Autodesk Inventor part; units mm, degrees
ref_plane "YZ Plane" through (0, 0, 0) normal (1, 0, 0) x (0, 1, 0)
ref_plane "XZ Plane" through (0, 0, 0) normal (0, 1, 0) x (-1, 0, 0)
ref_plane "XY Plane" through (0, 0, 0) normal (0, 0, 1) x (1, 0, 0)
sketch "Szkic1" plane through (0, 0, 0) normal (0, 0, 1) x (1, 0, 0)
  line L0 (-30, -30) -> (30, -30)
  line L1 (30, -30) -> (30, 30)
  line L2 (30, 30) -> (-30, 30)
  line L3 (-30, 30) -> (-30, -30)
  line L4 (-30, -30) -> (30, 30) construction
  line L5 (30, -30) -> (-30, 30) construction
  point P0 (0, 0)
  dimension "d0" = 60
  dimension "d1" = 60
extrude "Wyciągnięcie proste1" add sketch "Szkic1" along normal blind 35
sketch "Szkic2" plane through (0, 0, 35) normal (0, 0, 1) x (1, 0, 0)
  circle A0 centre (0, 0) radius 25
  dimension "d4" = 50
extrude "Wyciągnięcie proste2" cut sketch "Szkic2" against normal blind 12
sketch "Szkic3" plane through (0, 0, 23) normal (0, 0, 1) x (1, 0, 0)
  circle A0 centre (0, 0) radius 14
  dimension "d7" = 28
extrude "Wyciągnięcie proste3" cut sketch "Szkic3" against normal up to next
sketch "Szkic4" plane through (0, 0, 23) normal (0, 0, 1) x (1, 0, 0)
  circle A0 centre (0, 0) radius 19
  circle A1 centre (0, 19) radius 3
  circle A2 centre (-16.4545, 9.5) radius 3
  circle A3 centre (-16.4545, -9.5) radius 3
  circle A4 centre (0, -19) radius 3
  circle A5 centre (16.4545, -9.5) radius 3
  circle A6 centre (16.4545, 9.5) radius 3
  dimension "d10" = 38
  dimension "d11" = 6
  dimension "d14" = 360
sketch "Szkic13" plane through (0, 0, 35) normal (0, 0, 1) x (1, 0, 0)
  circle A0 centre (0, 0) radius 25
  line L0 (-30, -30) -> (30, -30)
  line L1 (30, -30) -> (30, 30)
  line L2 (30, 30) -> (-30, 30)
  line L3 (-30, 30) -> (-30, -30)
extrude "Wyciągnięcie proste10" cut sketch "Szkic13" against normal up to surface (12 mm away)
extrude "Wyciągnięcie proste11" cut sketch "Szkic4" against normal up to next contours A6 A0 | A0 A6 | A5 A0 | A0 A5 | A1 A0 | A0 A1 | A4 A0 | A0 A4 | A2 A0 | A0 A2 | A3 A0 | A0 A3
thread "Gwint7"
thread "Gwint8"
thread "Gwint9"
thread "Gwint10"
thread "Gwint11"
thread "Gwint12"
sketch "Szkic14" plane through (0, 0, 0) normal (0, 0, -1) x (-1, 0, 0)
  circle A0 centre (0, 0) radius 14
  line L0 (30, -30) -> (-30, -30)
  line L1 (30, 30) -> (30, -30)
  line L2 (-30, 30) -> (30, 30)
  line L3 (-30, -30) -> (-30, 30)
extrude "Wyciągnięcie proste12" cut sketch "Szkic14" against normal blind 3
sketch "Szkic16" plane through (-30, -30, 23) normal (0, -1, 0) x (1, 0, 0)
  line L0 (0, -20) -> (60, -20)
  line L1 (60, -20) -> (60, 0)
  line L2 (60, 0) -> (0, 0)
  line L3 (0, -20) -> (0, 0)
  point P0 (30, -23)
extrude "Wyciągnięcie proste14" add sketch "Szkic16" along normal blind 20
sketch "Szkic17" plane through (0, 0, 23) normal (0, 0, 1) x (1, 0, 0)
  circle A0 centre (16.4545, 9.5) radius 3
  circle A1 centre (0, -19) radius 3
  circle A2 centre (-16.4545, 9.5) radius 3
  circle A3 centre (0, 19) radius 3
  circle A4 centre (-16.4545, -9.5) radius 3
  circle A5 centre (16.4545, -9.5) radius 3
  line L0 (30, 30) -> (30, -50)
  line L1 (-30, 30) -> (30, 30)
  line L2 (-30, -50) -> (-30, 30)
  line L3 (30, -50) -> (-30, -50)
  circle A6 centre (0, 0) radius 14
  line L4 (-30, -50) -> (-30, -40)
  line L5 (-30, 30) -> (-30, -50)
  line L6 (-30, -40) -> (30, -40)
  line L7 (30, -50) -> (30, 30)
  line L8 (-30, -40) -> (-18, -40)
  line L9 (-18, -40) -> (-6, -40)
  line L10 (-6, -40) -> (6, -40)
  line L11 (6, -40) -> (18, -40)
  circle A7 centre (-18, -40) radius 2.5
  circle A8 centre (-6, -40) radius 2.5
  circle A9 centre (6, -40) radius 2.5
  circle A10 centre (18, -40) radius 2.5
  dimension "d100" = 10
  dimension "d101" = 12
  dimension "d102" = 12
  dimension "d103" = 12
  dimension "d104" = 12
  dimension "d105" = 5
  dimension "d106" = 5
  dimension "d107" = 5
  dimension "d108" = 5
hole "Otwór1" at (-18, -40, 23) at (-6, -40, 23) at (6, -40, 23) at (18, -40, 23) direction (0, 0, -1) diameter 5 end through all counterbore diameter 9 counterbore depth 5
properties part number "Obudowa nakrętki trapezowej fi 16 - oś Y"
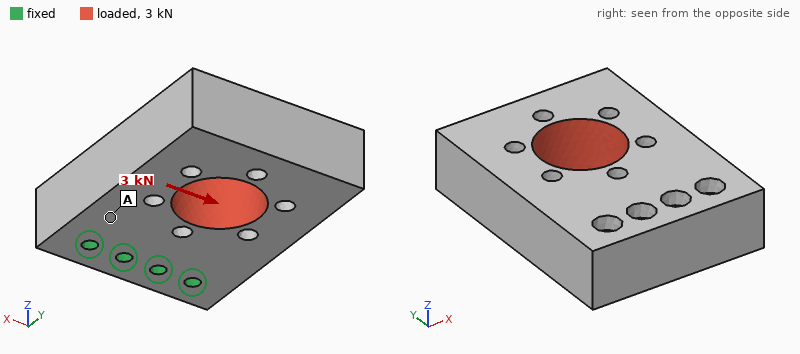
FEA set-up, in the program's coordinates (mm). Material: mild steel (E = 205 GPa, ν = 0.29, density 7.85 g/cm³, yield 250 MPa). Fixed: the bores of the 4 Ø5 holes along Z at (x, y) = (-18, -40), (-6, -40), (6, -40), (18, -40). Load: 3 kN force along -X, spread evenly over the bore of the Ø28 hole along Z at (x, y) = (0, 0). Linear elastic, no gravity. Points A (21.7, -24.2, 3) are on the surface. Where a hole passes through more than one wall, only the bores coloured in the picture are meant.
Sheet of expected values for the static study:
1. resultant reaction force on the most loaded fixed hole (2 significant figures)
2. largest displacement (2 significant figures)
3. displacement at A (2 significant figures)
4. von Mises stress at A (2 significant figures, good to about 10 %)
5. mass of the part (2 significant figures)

3.0 kN
8.5 µm
1.4 µm
5.3 MPa
610 g
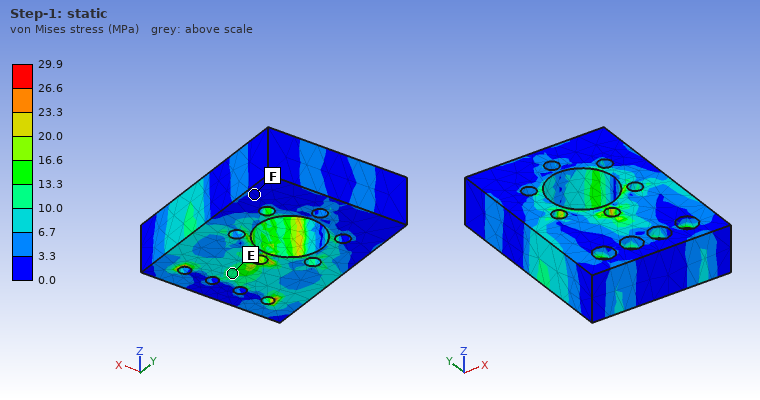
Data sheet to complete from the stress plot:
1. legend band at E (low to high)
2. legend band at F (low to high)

10.0 to 13.3 MPa
0.0 to 3.3 MPa
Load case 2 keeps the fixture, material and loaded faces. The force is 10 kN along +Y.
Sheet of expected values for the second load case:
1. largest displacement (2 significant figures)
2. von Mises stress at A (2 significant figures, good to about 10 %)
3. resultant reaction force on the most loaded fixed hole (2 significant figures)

6.2 µm
9.6 MPa
3.5 kN
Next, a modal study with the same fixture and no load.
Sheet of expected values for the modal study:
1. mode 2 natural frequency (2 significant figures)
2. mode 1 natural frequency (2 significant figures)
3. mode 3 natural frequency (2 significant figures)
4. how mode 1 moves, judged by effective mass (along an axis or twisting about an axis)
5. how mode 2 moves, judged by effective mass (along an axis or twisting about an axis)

5100 Hz
2700 Hz
5700 Hz
along Z
along X
